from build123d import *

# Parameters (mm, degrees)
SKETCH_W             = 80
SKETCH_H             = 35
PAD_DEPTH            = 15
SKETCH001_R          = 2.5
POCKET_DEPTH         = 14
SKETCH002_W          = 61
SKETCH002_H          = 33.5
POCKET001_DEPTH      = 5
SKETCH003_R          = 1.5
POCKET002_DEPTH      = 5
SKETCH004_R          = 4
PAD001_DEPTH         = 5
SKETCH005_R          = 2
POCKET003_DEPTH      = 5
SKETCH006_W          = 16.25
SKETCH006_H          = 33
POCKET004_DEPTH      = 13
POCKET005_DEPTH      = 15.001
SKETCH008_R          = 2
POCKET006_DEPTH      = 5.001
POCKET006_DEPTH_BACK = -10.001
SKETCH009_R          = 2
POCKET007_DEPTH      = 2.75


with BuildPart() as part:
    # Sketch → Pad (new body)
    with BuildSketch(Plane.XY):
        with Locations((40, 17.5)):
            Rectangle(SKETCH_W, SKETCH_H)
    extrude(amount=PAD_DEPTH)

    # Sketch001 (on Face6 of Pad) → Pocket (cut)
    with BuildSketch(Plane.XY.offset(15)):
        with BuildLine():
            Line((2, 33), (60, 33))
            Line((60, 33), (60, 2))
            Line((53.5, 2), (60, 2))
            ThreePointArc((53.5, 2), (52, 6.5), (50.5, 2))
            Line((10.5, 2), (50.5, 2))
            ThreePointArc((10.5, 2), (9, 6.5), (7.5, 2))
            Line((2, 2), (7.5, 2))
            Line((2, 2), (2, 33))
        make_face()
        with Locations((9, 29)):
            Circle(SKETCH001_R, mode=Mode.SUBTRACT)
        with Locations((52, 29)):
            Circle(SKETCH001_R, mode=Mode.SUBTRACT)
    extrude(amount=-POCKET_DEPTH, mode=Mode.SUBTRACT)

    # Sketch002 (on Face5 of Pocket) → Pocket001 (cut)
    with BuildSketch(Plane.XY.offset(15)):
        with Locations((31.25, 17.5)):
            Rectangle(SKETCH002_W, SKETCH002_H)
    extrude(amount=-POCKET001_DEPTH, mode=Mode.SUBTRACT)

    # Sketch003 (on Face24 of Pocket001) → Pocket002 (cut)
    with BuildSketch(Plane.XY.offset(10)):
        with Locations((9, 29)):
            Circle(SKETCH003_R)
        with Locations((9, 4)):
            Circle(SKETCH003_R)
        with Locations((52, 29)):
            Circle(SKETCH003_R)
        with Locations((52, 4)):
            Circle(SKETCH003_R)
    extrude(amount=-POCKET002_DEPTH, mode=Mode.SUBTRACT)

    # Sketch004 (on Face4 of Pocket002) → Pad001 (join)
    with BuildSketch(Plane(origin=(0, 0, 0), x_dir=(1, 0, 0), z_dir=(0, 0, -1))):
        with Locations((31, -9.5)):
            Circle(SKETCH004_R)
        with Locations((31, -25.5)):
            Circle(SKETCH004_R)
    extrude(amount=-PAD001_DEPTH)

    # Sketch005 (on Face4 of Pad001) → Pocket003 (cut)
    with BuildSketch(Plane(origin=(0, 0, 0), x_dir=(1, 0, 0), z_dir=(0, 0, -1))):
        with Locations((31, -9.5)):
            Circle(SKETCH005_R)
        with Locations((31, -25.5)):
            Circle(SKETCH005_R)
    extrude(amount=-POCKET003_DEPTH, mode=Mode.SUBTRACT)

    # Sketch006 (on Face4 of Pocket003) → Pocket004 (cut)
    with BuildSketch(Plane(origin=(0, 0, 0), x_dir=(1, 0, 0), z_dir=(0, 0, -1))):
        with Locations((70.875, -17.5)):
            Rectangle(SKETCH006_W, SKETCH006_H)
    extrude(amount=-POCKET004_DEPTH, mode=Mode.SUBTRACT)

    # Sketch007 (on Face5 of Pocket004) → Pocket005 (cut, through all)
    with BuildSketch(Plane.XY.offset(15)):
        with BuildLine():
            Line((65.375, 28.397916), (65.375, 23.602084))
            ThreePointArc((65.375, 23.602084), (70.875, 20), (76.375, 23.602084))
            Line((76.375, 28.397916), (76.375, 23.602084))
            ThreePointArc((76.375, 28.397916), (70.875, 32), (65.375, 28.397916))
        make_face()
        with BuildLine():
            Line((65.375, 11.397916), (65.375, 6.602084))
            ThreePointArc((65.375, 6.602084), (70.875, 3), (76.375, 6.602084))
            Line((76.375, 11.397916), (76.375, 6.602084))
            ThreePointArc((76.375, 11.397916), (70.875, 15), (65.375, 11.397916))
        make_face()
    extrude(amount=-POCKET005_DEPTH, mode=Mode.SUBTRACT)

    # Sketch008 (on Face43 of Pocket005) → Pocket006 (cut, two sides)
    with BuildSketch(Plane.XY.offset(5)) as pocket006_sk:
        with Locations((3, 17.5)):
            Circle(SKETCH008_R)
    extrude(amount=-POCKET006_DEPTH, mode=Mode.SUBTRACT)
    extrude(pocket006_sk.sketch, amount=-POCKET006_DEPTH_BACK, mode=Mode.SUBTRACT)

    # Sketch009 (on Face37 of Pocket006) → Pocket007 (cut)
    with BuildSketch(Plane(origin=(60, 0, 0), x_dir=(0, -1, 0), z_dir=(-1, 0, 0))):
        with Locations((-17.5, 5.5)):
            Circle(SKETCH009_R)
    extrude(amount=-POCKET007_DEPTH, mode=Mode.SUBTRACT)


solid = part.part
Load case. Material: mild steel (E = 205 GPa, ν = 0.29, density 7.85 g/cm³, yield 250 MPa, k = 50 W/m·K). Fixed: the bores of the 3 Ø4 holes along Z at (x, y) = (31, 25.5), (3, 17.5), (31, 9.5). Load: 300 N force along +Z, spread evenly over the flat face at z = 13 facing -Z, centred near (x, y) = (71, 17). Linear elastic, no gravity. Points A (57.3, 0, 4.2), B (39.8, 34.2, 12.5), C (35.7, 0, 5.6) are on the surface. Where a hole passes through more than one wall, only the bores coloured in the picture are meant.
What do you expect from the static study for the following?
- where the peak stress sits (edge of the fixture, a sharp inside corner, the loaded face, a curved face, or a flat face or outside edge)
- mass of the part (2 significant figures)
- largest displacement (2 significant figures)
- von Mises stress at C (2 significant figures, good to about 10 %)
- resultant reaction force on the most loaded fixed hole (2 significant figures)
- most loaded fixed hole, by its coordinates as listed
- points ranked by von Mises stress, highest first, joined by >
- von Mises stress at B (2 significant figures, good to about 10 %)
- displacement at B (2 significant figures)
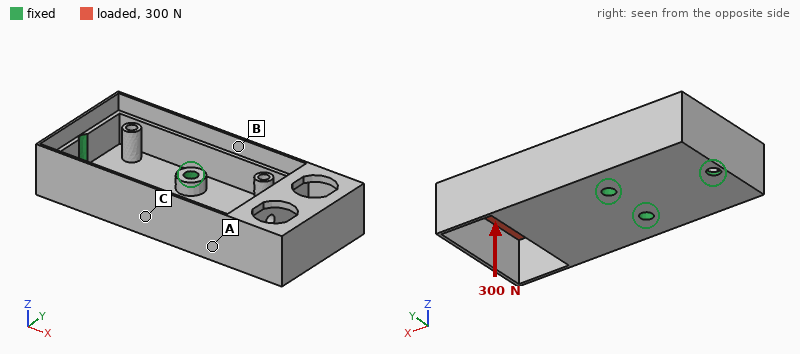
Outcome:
a flat face or outside edge
70 g
0.14 mm
31 MPa
380 N
(3, 17.5)
B > C > A
60 MPa
0.056 mm
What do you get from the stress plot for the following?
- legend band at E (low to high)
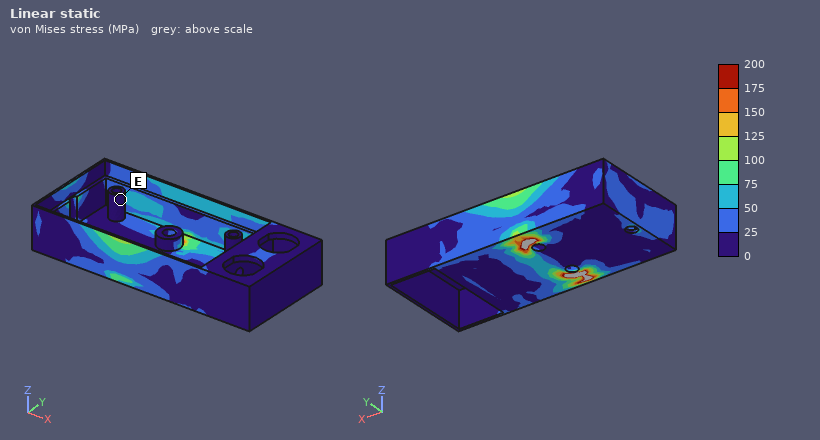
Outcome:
0 to 25 MPa
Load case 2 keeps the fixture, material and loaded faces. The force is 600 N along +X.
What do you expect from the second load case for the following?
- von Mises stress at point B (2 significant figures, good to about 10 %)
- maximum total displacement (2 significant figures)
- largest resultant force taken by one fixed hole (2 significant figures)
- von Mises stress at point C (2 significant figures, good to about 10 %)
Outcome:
44 MPa
73 µm
270 N
19 MPa
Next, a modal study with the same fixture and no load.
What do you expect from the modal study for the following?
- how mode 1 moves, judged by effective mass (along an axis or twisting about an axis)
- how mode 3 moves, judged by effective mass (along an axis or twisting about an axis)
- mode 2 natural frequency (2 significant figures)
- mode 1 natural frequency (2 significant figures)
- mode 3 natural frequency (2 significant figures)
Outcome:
along Z
along Y
1800 Hz
1600 Hz
5200 Hz
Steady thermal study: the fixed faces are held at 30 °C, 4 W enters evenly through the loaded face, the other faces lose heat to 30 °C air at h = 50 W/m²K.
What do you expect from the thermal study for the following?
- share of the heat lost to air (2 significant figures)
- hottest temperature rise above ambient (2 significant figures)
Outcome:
84 %
20 K
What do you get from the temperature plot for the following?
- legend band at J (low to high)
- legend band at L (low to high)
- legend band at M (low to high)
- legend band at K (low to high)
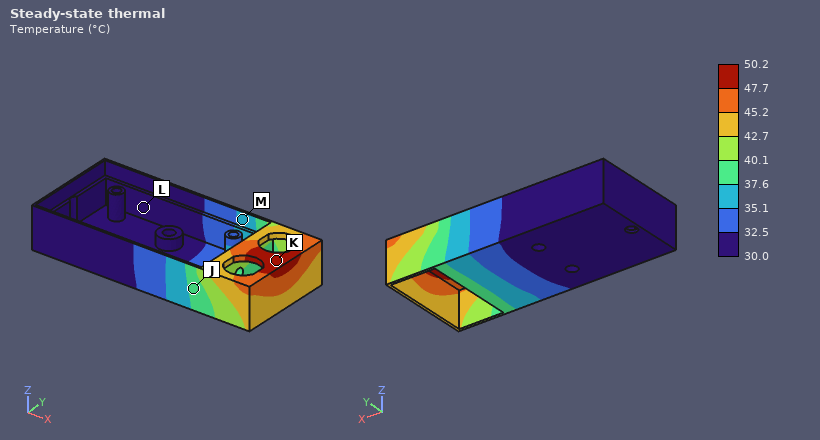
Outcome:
37.6 to 40.1 °C
30.0 to 32.5 °C
35.1 to 37.6 °C
47.7 to 50.2 °C
